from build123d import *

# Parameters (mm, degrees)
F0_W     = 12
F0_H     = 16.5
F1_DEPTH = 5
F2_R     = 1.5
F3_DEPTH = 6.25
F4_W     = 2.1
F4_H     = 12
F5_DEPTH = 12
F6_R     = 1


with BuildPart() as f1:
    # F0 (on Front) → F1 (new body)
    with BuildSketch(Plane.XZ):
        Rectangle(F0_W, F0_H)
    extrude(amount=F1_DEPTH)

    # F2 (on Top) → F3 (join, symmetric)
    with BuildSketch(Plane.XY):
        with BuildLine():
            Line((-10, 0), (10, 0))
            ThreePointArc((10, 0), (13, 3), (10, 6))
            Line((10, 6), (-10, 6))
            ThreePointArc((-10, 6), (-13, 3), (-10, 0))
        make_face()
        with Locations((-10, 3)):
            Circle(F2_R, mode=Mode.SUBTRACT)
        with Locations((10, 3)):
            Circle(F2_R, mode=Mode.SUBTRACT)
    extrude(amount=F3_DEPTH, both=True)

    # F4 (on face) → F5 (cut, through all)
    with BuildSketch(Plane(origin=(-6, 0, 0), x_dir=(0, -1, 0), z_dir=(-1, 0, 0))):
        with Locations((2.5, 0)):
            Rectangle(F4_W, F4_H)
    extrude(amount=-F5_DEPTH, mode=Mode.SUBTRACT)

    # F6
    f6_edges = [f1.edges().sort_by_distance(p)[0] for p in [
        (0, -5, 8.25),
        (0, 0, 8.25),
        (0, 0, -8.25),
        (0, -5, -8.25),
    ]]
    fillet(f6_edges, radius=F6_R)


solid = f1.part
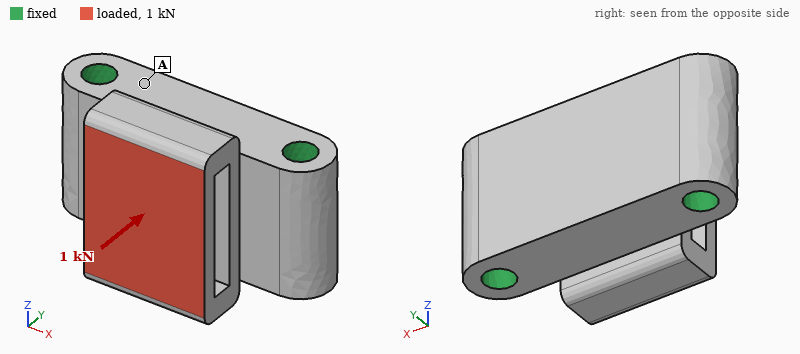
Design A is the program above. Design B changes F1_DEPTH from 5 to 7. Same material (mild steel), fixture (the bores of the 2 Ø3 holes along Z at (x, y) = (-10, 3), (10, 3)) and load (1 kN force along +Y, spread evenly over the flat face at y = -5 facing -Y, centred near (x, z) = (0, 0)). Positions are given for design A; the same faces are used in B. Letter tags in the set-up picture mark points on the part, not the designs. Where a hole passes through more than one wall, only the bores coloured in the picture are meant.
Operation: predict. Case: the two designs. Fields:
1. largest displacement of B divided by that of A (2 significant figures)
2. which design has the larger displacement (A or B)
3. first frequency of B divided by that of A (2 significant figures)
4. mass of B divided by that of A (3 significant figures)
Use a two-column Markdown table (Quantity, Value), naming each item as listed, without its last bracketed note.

| Quantity | Value |
|---|---|
| largest displacement of B divided by that of A | 0.34 |
| which design has the larger displacement | A |
| first frequency of B divided by that of A | 0.76 |
| mass of B divided by that of A | 1.17 |
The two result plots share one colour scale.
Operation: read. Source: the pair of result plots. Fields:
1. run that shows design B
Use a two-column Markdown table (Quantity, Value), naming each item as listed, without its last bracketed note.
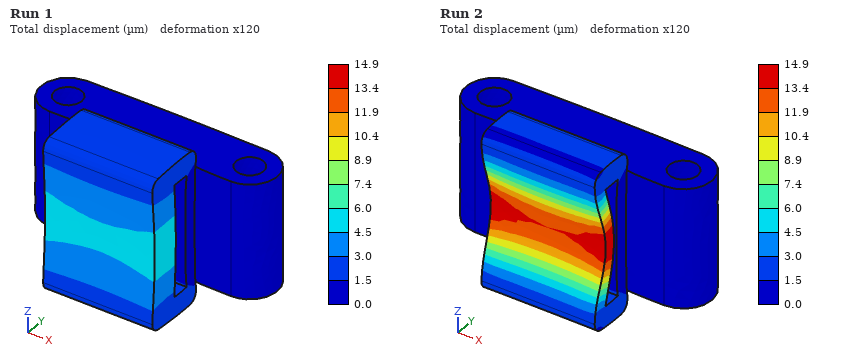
| Quantity | Value |
|---|---|
| run that shows design B | Run 1 |
